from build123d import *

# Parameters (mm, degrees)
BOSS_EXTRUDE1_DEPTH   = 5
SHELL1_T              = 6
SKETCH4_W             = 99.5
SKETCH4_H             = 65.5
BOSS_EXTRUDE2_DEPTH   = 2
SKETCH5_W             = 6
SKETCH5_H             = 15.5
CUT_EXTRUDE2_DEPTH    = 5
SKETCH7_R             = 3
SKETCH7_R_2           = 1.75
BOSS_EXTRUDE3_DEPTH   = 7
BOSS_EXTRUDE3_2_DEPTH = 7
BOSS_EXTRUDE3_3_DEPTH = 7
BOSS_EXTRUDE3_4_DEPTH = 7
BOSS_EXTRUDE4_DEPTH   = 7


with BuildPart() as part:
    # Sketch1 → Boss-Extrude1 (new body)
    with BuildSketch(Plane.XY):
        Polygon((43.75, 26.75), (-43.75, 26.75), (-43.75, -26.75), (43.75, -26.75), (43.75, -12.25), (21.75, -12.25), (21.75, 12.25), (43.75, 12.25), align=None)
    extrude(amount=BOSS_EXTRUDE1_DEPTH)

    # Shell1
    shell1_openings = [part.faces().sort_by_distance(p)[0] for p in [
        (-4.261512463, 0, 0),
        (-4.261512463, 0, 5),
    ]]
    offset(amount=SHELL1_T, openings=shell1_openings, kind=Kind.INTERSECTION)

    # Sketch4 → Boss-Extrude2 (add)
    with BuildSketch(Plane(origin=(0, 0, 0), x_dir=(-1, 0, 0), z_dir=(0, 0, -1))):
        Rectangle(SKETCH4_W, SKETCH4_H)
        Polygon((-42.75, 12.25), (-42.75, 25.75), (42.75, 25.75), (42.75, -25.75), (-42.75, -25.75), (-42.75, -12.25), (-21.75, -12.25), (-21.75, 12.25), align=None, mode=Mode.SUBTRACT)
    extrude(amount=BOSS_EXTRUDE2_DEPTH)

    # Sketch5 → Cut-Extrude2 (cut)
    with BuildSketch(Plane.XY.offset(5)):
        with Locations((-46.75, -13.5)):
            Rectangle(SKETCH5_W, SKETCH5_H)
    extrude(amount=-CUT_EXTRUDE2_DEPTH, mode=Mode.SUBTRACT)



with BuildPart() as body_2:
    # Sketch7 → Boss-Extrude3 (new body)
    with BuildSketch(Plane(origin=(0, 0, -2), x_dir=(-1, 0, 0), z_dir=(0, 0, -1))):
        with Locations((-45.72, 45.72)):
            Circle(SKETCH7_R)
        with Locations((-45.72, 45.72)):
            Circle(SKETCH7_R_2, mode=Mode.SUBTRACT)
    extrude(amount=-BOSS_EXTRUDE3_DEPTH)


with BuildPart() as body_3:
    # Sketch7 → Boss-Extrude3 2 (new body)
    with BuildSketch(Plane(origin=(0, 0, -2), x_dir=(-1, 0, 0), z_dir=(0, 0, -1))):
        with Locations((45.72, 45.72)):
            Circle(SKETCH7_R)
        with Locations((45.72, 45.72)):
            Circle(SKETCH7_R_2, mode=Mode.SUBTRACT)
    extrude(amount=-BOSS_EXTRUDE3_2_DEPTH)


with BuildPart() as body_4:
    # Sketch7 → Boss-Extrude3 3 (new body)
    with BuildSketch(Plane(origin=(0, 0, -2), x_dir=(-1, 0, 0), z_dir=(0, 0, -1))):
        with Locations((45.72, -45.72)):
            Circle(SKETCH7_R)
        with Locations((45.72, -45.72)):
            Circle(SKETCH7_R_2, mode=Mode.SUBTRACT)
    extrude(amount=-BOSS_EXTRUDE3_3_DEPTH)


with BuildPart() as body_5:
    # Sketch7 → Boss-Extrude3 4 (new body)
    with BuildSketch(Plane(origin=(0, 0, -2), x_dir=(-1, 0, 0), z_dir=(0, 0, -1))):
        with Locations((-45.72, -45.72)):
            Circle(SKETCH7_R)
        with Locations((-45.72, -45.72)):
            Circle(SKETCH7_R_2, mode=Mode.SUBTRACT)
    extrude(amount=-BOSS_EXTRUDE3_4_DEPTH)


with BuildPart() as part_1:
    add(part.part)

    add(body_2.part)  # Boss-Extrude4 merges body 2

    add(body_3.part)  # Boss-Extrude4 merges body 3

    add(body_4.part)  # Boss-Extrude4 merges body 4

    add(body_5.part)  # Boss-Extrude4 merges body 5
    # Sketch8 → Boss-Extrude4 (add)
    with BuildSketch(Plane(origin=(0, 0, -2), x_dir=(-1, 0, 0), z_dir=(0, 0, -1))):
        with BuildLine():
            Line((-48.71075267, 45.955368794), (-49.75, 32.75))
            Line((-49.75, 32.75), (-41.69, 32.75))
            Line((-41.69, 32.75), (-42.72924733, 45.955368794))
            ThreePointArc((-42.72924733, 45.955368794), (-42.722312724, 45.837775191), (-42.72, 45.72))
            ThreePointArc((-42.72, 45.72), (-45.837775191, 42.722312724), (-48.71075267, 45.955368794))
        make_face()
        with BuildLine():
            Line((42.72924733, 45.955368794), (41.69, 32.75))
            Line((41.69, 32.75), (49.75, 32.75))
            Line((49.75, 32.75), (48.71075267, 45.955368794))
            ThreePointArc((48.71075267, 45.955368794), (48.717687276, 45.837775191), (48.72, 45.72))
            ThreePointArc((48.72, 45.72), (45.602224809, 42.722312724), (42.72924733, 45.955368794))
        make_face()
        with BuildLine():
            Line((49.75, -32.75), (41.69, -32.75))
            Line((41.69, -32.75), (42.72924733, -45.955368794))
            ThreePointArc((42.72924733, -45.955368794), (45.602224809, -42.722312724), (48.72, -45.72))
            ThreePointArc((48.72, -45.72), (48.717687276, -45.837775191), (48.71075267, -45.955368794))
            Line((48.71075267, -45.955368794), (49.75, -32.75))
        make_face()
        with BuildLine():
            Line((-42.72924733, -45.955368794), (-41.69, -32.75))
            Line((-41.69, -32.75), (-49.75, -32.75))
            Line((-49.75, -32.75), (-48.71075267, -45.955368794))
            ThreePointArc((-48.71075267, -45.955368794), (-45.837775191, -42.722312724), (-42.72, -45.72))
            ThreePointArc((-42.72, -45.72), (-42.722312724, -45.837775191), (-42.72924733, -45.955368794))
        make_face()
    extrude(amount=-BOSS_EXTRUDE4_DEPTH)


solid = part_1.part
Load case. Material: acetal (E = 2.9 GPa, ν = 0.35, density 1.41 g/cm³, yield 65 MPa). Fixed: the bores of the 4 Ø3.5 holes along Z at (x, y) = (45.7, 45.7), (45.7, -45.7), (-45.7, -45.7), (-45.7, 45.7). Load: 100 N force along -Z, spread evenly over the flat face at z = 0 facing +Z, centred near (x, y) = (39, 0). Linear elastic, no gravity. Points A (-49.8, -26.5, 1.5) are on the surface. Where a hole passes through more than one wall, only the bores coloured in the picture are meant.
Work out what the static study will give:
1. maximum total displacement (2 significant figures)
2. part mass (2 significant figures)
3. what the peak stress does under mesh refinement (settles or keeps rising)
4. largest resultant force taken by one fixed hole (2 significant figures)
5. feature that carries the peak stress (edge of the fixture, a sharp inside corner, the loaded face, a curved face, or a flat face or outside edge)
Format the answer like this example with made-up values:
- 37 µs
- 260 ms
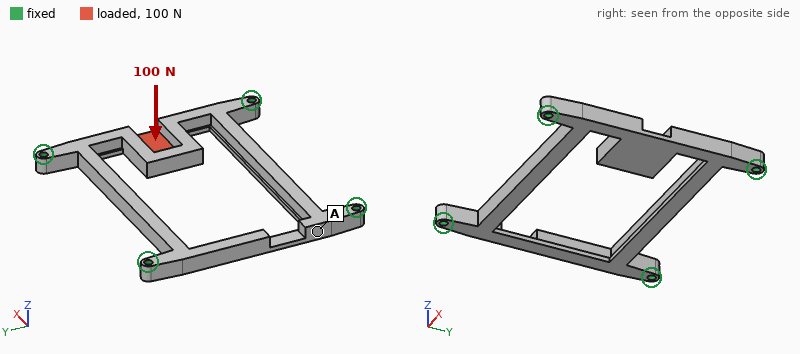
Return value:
- 1.6 mm
- 25 g
- keeps rising
- 130 N
- edge of the fixture
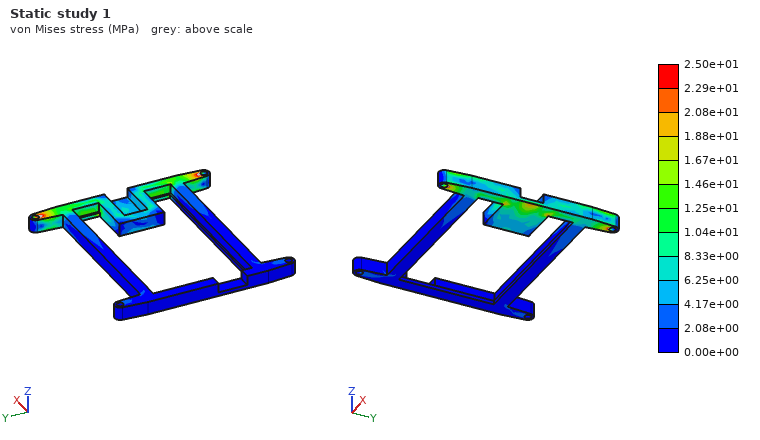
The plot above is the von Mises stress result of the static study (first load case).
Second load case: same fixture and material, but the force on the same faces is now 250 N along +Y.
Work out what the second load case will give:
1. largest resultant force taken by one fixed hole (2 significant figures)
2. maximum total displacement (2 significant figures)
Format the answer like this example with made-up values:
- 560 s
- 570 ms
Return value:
- 130 N
- 0.29 mm
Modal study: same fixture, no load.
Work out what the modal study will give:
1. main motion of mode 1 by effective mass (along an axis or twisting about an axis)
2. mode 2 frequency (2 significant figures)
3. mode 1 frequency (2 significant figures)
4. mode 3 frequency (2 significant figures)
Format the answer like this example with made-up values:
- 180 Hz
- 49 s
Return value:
- along Z
- 830 Hz
- 550 Hz
- 850 Hz
